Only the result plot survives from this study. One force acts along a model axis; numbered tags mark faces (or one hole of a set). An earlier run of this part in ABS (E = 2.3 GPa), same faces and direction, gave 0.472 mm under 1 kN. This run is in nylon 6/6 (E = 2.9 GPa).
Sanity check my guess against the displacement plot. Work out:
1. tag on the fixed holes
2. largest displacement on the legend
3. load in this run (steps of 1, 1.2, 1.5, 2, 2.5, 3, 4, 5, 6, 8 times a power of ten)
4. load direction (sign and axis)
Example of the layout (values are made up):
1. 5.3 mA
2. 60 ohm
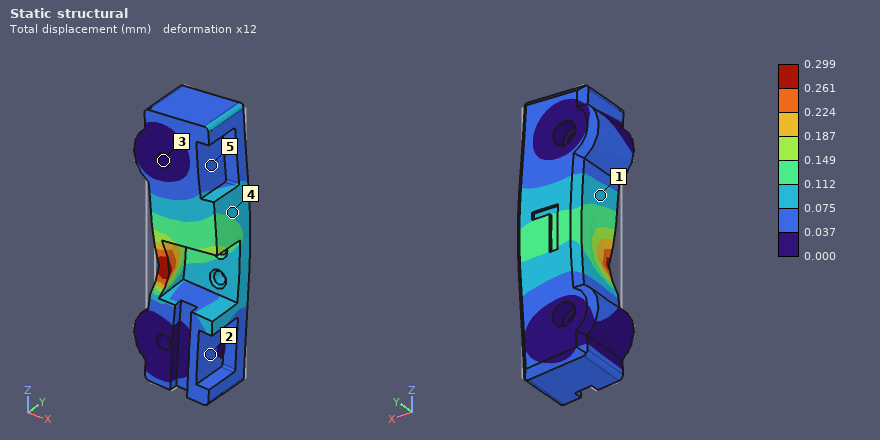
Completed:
1. 3
2. 0.299 mm
3. 800 N
4. +X
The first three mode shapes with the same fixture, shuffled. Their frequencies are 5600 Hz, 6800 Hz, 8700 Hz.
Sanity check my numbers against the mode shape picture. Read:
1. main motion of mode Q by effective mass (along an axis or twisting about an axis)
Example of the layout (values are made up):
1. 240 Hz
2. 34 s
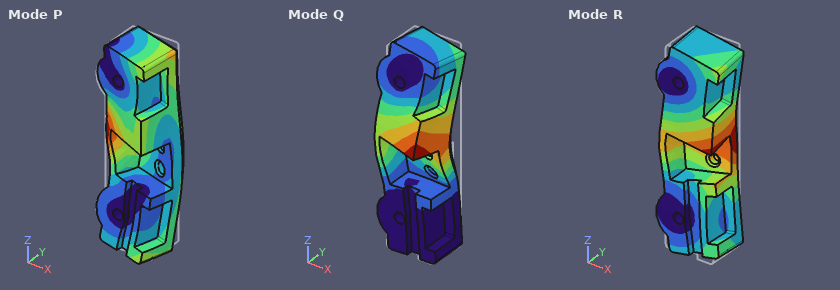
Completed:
1. along Y
